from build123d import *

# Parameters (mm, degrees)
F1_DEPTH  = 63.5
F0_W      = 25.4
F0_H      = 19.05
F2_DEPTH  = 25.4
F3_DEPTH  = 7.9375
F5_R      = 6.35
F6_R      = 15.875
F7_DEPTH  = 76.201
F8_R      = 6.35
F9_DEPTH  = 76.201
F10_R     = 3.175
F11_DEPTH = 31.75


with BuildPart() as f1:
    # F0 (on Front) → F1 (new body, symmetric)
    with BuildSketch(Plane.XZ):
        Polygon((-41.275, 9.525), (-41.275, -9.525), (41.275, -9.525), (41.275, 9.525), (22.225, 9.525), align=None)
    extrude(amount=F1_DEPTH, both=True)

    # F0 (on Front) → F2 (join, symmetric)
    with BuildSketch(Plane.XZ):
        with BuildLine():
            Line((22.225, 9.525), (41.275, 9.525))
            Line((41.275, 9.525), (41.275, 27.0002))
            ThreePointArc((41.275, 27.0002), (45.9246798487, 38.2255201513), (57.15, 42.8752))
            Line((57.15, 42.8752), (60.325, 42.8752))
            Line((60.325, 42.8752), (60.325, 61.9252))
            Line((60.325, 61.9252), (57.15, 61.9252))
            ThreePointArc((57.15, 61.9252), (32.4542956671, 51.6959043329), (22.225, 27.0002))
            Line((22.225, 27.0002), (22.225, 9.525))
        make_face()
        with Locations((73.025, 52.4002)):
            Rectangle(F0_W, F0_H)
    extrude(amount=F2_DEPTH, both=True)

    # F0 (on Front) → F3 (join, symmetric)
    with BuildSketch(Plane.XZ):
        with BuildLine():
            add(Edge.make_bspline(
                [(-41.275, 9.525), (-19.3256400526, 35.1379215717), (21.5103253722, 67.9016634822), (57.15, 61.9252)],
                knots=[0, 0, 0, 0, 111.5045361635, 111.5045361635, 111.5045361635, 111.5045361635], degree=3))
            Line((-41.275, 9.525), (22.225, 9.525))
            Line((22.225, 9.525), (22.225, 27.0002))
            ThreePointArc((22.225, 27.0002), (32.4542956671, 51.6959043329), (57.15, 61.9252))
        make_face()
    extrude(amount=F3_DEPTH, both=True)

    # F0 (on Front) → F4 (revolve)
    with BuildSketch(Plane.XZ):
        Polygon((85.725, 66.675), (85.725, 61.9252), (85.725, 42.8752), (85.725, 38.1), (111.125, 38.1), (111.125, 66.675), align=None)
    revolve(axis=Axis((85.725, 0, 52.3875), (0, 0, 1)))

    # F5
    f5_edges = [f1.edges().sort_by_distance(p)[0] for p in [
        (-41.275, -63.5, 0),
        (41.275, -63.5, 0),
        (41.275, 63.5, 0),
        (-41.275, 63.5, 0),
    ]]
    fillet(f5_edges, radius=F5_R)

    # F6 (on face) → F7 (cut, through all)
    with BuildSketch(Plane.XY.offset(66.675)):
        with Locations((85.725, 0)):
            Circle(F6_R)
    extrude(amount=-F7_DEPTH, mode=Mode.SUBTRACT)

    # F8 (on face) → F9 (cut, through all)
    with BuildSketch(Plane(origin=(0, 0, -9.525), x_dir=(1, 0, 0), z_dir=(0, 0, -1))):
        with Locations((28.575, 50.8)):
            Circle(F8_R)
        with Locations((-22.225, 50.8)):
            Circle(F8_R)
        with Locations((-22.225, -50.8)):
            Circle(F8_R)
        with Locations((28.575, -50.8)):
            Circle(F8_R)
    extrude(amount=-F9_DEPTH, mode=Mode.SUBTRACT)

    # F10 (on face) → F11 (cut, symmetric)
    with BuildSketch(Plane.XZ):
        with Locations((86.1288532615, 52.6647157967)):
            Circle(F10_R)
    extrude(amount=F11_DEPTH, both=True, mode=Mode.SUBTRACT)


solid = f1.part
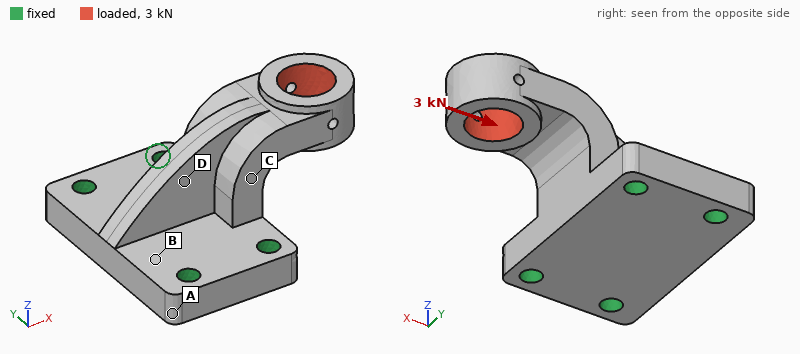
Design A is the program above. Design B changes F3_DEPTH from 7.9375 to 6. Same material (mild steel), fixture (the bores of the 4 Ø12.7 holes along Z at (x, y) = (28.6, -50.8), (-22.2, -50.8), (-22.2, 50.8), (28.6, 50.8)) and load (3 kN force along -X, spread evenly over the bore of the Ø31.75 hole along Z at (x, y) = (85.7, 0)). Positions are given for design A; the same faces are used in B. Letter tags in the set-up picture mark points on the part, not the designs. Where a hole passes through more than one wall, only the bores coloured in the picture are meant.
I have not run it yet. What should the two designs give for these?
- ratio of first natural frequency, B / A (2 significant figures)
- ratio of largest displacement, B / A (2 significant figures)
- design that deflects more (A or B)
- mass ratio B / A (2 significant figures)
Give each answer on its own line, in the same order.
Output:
0.97
1.1
B
0.98
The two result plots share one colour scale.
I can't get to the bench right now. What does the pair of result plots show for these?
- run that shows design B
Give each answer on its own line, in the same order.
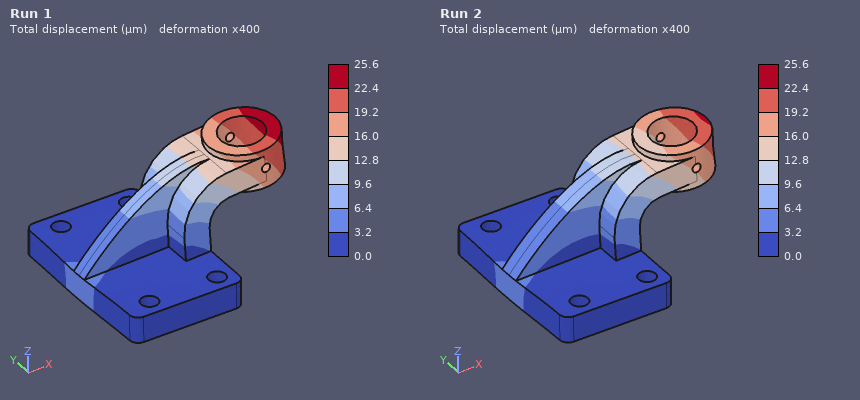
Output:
Run 1
